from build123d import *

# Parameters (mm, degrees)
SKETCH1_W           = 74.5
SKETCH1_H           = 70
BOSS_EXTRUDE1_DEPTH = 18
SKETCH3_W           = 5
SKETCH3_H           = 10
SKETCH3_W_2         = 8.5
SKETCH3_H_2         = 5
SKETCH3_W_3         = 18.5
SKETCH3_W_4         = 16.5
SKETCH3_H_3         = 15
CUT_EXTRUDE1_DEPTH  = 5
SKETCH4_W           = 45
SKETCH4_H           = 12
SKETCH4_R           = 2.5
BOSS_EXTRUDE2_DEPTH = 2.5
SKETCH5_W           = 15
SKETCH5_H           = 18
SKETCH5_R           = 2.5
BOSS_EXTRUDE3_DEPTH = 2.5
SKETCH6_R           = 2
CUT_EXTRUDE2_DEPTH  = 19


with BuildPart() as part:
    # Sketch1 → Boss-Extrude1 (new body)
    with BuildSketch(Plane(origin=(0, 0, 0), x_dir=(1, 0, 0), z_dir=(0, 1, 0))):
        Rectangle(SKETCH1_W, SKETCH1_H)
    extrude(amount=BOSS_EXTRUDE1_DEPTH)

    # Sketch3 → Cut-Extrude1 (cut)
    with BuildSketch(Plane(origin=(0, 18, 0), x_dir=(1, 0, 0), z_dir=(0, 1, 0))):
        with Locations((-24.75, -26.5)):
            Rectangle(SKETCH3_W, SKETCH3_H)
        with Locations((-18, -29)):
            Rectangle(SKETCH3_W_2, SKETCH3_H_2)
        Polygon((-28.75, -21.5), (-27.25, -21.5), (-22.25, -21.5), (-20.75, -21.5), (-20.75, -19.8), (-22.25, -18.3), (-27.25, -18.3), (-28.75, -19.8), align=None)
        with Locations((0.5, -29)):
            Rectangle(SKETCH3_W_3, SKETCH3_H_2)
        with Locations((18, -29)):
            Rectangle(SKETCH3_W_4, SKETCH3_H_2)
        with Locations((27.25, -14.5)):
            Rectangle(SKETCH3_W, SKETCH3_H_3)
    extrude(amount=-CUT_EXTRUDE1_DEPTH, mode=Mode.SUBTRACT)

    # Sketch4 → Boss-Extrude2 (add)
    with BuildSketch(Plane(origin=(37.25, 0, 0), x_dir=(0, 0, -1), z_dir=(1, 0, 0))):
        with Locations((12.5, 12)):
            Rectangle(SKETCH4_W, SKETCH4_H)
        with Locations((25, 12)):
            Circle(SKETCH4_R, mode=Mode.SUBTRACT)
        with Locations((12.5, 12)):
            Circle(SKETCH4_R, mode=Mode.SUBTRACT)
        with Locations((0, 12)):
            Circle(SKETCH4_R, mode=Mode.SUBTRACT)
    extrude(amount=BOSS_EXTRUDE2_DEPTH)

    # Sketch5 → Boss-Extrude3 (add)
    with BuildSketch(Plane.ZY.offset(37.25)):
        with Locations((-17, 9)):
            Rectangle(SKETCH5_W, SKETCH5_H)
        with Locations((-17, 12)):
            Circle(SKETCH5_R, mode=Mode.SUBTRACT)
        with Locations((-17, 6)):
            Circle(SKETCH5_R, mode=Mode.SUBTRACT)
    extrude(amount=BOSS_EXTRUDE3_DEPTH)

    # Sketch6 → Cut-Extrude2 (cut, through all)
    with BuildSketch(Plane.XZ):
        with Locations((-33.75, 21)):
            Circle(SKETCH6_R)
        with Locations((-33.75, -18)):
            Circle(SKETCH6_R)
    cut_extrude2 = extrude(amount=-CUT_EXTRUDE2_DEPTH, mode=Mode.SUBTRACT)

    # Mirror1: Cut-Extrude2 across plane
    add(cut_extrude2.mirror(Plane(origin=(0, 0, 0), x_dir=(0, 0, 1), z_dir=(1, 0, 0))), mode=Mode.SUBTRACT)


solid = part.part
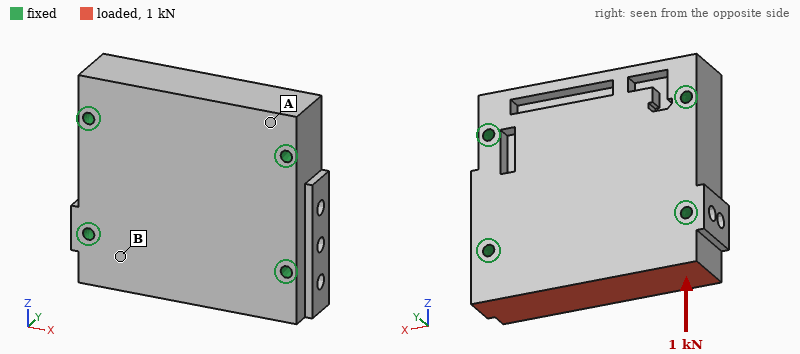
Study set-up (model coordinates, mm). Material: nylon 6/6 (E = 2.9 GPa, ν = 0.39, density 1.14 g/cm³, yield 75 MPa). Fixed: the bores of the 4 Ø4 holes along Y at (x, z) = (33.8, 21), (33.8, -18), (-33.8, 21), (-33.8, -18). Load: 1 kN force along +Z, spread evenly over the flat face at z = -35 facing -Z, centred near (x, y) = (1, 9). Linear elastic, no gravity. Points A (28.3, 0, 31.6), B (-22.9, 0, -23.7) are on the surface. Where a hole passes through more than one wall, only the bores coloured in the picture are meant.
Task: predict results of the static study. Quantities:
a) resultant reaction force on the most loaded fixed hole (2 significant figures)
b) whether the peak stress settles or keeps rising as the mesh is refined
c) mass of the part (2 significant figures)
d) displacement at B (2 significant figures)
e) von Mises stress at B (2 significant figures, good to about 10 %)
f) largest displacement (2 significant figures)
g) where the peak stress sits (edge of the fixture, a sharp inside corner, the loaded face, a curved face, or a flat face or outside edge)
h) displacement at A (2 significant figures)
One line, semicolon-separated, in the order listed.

370 N; keeps rising; 110 g; 7.8 µm; 0.67 MPa; 15 µm; edge of the fixture; 3.2 µm
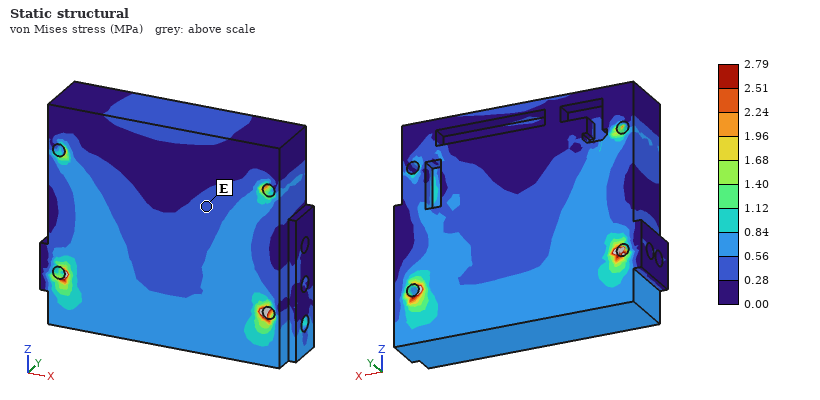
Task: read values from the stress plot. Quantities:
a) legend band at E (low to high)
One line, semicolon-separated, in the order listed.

0.28 to 0.56 MPa
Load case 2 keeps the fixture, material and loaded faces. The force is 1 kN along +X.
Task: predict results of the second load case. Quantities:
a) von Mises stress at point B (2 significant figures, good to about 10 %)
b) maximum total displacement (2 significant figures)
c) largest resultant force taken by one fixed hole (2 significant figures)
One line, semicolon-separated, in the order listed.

1.7 MPa; 28 µm; 510 N
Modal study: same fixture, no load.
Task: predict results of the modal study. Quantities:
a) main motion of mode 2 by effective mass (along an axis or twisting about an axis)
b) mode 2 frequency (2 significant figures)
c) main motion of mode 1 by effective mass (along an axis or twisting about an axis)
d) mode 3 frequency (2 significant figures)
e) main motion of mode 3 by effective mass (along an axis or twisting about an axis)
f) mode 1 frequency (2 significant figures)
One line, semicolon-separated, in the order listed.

twisting about X; 4200 Hz; along Y; 5400 Hz; along Z; 3500 Hz
